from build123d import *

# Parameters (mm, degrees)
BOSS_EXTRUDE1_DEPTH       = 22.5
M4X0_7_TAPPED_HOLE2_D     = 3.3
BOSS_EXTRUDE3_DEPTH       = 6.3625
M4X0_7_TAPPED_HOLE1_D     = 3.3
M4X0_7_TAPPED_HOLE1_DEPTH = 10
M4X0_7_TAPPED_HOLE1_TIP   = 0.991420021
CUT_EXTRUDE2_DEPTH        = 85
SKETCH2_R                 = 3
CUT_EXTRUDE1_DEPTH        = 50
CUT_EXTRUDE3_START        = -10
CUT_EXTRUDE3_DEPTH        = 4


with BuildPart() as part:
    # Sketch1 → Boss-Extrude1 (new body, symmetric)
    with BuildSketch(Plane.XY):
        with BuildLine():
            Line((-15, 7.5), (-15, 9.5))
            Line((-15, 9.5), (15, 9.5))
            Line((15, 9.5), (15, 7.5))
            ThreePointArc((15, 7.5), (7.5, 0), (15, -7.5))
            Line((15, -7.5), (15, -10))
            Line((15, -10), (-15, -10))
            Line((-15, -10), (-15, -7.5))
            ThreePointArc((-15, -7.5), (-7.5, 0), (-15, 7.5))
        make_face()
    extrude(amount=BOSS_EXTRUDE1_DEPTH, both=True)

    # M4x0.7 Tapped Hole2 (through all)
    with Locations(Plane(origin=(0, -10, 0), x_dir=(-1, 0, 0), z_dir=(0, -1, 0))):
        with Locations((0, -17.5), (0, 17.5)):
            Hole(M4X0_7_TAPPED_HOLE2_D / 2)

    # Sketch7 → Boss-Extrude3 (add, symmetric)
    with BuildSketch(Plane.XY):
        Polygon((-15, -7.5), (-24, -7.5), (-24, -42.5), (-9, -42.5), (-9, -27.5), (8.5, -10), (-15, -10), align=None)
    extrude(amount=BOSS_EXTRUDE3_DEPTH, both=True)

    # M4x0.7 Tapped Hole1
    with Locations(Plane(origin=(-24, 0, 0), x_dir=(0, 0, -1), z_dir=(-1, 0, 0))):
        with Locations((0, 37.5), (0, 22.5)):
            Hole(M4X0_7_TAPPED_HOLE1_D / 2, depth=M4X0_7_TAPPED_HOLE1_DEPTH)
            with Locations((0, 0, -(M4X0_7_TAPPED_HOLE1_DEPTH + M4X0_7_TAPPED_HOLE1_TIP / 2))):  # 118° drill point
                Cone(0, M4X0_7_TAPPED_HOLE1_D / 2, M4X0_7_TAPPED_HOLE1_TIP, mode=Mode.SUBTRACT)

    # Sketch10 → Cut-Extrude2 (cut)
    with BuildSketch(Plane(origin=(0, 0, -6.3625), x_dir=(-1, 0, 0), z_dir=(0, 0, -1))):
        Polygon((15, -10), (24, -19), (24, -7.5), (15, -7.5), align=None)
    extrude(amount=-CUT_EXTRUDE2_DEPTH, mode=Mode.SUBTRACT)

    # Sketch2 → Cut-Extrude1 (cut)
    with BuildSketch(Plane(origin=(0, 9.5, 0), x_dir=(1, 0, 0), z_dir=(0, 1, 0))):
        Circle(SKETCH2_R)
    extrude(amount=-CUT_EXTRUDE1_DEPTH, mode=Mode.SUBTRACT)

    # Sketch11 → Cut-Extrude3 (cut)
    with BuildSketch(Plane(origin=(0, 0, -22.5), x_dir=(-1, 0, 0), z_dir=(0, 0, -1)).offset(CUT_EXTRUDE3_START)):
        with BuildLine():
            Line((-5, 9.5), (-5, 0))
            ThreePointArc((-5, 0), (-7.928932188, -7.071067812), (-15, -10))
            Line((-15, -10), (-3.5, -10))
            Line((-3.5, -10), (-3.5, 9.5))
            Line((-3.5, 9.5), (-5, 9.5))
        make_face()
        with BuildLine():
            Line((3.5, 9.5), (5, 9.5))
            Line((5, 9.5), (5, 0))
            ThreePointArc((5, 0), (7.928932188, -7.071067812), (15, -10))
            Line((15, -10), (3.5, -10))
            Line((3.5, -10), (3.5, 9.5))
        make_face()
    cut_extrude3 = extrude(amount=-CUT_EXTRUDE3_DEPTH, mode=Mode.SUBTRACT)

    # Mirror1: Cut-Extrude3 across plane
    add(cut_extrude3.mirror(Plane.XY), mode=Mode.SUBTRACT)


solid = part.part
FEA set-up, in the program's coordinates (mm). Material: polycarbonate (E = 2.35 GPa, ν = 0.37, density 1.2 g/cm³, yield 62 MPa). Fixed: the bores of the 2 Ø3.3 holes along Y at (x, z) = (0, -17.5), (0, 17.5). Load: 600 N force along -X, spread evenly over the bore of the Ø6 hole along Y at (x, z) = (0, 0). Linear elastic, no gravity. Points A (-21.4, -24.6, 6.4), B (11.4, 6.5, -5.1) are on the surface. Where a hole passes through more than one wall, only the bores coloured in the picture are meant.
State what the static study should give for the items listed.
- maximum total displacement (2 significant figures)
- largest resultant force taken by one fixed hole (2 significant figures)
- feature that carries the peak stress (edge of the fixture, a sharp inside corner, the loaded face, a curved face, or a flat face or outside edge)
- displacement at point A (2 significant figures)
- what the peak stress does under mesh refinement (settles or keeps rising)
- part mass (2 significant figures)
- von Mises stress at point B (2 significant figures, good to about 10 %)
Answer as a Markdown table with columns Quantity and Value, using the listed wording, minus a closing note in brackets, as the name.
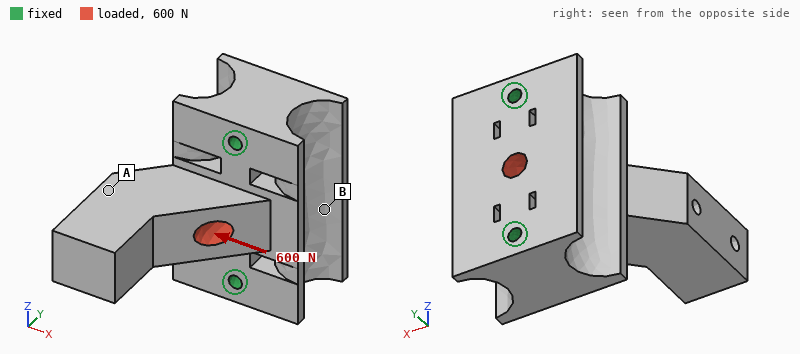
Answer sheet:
| Quantity | Value |
|---|---|
| maximum total displacement | 0.18 mm |
| largest resultant force taken by one fixed hole | 300 N |
| feature that carries the peak stress | edge of the fixture |
| displacement at point A | 0.12 mm |
| what the peak stress does under mesh refinement | keeps rising |
| part mass | 29 g |
| von Mises stress at point B | 2.1 MPa |
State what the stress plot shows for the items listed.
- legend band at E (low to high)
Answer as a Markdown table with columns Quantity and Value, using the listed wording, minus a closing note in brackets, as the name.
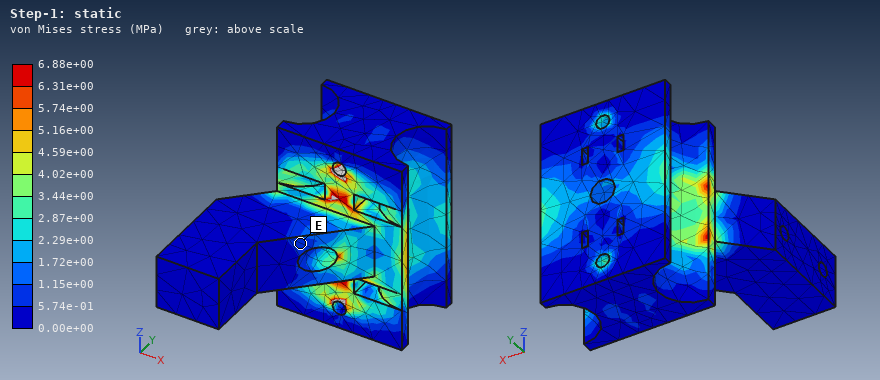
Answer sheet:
| Quantity | Value |
|---|---|
| legend band at E | 5.74e-01 to 1.15e+00 MPa |
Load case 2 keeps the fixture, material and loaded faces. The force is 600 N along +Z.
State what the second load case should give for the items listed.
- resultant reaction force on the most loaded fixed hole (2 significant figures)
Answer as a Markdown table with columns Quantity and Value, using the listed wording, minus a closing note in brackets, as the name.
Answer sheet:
| Quantity | Value |
|---|---|
| resultant reaction force on the most loaded fixed hole | 310 N |
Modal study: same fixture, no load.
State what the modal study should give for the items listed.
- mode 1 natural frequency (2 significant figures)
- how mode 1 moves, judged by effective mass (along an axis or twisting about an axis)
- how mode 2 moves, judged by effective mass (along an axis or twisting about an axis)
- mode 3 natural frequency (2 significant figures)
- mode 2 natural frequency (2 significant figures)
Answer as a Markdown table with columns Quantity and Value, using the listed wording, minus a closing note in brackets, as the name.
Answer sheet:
| Quantity | Value |
|---|---|
| mode 1 natural frequency | 1400 Hz |
| how mode 1 moves, judged by effective mass | along X |
| how mode 2 moves, judged by effective mass | along Z |
| mode 3 natural frequency | 4900 Hz |
| mode 2 natural frequency | 1700 Hz |
